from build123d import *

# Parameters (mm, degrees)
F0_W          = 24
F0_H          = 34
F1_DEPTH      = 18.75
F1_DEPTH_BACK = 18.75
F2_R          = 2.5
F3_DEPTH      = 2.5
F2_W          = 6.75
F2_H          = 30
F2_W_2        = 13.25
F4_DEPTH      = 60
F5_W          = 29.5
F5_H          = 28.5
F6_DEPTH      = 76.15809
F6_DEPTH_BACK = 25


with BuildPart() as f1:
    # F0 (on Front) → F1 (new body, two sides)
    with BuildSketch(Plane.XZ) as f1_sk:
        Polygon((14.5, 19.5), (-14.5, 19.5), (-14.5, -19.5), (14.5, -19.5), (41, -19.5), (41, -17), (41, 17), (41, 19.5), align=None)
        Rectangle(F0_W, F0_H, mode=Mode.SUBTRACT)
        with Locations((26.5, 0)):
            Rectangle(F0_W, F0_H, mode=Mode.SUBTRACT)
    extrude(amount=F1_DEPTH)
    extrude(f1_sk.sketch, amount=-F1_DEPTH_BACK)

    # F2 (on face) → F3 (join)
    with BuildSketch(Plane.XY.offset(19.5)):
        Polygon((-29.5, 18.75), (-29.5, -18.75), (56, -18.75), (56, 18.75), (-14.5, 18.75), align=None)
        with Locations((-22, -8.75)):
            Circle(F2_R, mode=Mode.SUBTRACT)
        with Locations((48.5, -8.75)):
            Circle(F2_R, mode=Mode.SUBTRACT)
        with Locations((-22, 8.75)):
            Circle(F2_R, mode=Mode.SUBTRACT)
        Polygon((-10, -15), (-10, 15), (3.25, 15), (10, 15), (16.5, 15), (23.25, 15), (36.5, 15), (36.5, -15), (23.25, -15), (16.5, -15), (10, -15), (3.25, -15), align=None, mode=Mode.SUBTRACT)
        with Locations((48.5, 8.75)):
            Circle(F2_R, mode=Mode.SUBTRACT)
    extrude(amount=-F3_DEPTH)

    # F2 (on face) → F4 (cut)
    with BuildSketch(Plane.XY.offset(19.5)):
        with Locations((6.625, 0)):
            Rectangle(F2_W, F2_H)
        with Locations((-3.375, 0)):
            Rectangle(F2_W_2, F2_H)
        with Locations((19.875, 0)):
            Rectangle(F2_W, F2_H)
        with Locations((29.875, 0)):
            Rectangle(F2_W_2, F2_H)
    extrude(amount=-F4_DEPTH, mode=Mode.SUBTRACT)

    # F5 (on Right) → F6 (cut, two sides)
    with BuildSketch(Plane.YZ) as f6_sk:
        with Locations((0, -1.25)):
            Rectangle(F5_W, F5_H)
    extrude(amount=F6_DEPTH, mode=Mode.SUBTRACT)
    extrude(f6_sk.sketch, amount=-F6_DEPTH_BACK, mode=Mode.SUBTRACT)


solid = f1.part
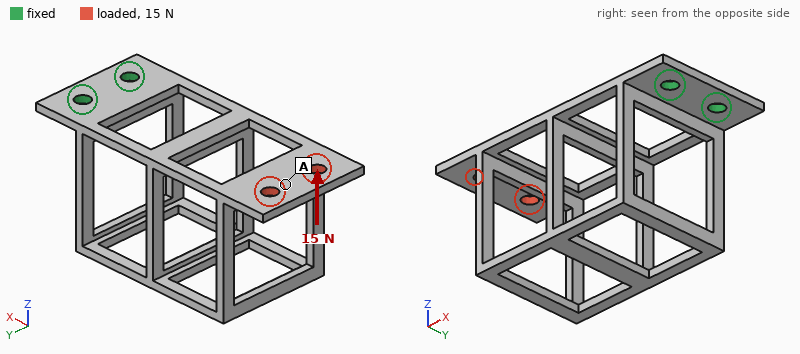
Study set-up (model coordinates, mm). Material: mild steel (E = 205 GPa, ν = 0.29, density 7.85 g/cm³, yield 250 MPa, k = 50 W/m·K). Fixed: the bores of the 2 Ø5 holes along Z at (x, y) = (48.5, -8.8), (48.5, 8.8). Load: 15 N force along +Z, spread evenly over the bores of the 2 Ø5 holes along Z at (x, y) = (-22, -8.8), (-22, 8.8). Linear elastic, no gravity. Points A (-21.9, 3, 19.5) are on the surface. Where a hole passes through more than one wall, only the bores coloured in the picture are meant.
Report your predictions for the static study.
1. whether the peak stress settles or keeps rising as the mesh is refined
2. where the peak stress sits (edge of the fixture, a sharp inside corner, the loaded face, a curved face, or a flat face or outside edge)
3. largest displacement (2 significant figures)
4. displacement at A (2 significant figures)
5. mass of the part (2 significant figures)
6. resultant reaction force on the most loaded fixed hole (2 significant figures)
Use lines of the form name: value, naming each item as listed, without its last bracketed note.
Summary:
whether the peak stress settles or keeps rising as the mesh is refined: keeps rising
where the peak stress sits: a sharp inside corner
largest displacement: 0.20 mm
displacement at A: 0.17 mm
mass of the part: 81 g
resultant reaction force on the most loaded fixed hole: 11 N
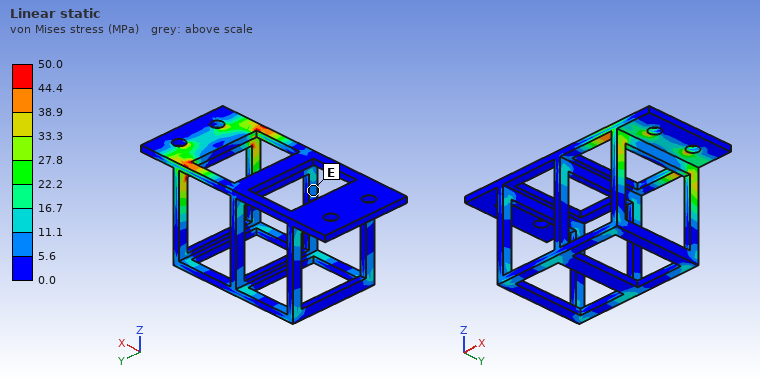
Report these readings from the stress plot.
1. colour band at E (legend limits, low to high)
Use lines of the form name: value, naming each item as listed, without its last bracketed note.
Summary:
colour band at E: 5.6 to 11.1 MPa
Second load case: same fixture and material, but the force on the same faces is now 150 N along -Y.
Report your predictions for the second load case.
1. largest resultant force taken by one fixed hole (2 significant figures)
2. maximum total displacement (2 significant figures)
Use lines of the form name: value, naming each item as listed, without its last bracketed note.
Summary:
largest resultant force taken by one fixed hole: 460 N
maximum total displacement: 0.12 mm
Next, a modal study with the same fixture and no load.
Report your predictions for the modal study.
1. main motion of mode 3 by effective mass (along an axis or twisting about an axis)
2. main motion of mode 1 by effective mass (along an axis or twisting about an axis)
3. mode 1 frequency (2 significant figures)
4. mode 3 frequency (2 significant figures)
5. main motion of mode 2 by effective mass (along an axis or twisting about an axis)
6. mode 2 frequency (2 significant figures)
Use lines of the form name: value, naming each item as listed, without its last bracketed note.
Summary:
main motion of mode 3 by effective mass: along Y
main motion of mode 1 by effective mass: along Z
mode 1 frequency: 250 Hz
mode 3 frequency: 1200 Hz
main motion of mode 2 by effective mass: along Y
mode 2 frequency: 800 Hz
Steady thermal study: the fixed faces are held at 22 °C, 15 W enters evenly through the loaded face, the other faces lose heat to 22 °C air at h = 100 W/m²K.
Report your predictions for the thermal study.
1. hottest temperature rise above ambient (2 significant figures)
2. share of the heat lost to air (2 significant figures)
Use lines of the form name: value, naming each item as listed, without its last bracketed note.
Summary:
hottest temperature rise above ambient: 73 K
share of the heat lost to air: 99 %
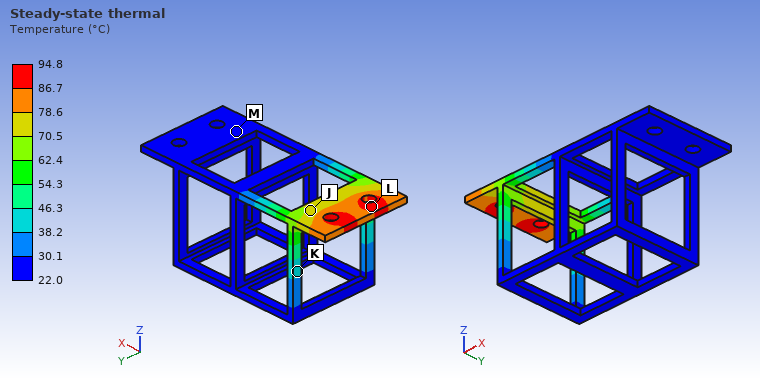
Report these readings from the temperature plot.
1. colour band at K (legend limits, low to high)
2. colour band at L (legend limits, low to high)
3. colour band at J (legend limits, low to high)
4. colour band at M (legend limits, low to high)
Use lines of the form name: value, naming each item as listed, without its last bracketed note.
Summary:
colour band at K: 38.2 to 46.3 °C
colour band at L: 86.7 to 94.8 °C
colour band at J: 70.5 to 78.6 °C
colour band at M: 22.0 to 30.1 °C
